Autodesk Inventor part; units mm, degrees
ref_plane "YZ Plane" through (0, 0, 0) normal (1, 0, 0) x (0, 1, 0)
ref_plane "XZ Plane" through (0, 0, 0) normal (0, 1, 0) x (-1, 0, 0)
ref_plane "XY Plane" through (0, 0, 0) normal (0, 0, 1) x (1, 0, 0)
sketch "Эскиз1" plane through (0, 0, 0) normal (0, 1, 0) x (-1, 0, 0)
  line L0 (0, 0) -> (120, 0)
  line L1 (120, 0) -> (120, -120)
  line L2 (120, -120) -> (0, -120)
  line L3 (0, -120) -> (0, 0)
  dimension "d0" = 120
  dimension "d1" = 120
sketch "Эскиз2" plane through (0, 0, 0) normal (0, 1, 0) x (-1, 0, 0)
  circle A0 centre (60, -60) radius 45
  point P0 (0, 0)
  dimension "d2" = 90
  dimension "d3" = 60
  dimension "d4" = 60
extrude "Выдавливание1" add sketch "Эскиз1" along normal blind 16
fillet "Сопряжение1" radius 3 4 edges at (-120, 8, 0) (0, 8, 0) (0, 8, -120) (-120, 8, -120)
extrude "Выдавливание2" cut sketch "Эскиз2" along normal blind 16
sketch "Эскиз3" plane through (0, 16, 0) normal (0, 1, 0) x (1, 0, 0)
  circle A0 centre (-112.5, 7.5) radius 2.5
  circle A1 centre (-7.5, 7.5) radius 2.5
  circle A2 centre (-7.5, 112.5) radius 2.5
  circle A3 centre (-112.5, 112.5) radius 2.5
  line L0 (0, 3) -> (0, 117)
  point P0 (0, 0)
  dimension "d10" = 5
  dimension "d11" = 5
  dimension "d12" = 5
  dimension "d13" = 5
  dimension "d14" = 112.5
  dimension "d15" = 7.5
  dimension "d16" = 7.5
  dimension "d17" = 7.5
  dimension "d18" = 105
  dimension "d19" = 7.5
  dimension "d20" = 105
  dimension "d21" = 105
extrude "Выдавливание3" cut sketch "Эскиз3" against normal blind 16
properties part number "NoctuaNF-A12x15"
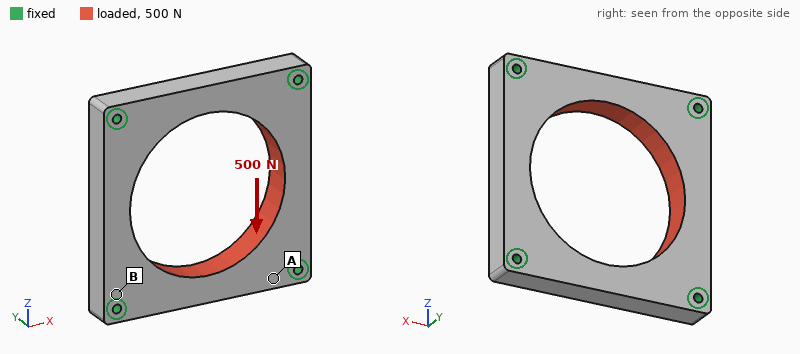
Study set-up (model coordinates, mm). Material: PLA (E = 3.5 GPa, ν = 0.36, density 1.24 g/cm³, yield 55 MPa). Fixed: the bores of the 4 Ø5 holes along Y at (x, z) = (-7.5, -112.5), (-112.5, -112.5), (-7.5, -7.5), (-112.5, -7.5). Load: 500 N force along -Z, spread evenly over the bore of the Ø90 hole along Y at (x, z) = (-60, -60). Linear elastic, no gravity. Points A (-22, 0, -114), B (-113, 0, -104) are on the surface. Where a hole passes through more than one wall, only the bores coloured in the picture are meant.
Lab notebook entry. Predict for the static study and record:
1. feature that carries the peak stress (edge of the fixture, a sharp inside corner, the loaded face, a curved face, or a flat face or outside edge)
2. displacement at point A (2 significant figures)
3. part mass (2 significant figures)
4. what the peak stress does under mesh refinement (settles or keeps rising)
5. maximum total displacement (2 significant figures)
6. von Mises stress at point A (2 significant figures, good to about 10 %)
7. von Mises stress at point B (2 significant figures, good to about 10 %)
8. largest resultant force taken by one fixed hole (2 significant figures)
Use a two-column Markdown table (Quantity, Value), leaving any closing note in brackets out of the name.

| Quantity | Value |
|---|---|
| feature that carries the peak stress | edge of the fixture |
| displacement at point A | 5.5 µm |
| part mass | 160 g |
| what the peak stress does under mesh refinement | keeps rising |
| maximum total displacement | 19 µm |
| von Mises stress at point A | 0.16 MPa |
| von Mises stress at point B | 0.57 MPa |
| largest resultant force taken by one fixed hole | 130 N |
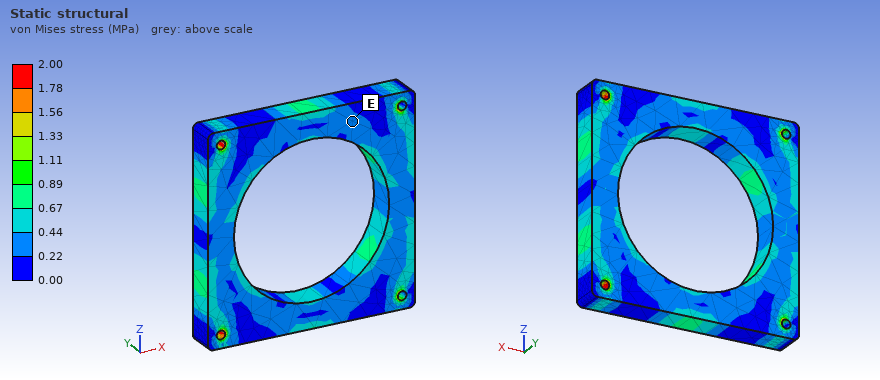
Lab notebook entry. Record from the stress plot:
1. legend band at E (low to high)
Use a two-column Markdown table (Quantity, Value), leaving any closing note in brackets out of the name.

| Quantity | Value |
|---|---|
| legend band at E | 0.22 to 0.44 MPa |
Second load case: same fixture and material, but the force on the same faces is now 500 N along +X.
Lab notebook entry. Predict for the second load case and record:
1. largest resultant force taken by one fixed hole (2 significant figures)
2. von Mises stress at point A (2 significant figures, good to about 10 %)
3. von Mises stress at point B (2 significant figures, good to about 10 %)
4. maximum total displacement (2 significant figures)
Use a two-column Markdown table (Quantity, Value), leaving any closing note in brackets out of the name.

| Quantity | Value |
|---|---|
| largest resultant force taken by one fixed hole | 130 N |
| von Mises stress at point A | 0.47 MPa |
| von Mises stress at point B | 0.26 MPa |
| maximum total displacement | 19 µm |
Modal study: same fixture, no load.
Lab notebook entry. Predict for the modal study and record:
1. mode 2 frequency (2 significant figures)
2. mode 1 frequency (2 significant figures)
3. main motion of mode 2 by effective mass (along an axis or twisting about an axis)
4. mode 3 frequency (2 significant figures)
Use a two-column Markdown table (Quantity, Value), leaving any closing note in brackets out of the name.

| Quantity | Value |
|---|---|
| mode 2 frequency | 2000 Hz |
| mode 1 frequency | 1500 Hz |
| main motion of mode 2 by effective mass | along Y |
| mode 3 frequency | 2200 Hz |
